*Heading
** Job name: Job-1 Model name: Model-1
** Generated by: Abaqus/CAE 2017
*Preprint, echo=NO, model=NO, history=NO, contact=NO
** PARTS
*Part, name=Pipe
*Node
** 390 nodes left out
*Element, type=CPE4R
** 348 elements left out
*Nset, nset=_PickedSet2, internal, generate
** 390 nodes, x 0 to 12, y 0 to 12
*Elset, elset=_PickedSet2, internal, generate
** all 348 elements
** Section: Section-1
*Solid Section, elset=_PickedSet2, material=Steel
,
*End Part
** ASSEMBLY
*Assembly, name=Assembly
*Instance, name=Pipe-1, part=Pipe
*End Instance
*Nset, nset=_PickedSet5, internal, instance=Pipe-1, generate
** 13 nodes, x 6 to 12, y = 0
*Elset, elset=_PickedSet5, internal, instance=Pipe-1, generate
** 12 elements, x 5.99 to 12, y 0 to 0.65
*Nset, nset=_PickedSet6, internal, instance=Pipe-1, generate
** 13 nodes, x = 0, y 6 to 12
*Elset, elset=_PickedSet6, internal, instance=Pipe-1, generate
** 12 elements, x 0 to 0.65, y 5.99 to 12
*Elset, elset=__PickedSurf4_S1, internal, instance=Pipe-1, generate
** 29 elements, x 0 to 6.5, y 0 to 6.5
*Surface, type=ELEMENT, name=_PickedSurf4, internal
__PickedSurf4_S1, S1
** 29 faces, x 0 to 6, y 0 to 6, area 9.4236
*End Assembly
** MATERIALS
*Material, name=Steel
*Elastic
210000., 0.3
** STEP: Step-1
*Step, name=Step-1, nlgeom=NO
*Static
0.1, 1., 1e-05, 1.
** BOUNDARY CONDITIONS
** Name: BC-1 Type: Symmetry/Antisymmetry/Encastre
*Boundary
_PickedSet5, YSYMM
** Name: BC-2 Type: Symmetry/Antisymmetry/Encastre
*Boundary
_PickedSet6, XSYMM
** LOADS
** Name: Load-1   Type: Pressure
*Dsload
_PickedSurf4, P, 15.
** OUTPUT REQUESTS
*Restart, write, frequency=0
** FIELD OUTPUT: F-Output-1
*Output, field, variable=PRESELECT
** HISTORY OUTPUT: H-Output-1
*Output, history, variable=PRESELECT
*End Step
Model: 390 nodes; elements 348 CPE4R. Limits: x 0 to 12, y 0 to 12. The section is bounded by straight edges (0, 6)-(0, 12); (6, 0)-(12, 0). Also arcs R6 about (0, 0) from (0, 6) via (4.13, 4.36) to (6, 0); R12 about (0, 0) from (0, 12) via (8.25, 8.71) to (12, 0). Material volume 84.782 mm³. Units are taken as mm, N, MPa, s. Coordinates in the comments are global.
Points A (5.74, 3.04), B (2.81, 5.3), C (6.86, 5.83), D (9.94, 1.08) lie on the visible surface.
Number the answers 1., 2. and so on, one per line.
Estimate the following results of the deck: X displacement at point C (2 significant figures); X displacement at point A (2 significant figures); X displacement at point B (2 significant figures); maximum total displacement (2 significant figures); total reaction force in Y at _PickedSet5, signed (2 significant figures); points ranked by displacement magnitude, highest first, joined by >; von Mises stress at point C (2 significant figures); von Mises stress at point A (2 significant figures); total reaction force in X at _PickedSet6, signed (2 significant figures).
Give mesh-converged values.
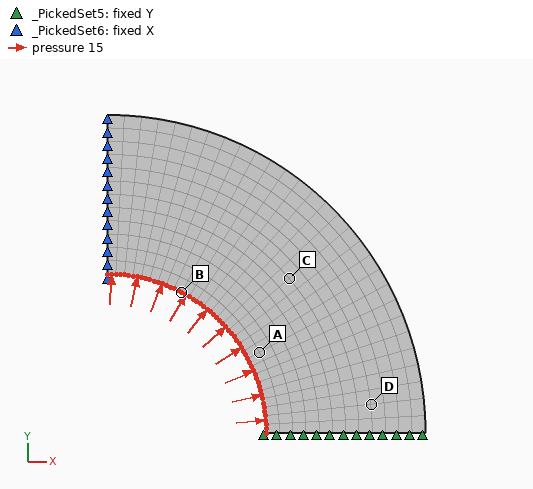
1. 4.6e-04 mm
2. 6.8e-04 mm
3. 3.8e-04 mm
4. 8.2e-04 mm
5. -90 N
6. B > A > C > D
7. 16 MPa
8. 30 MPa
9. -90 N
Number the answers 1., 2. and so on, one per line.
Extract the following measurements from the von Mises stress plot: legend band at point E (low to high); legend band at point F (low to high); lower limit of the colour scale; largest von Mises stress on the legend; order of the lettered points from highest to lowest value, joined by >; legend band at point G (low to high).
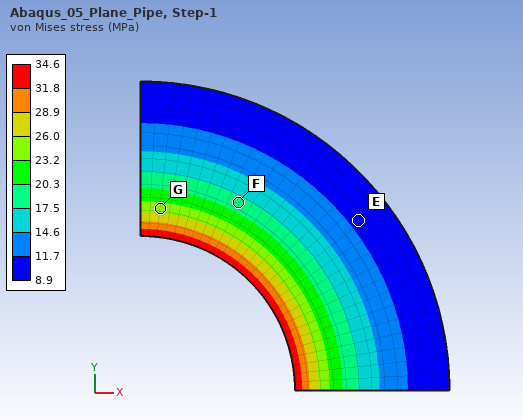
1. 8.9 to 11.7 MPa
2. 17.5 to 20.3 MPa
3. 8.9 MPa
4. 34.6 MPa
5. G > F > E
6. 23.2 to 26.0 MPa
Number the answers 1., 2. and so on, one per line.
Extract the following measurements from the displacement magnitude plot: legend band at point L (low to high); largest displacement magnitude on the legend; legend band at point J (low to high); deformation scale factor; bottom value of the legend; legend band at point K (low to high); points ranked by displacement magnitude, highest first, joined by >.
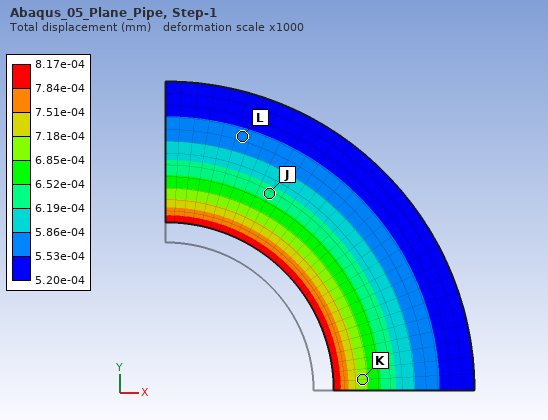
1. 5.53e-04 to 5.86e-04 mm
2. 8.17e-04 mm
3. 6.19e-04 to 6.52e-04 mm
4. 1000
5. 5.20e-04 mm
6. 6.85e-04 to 7.18e-04 mm
7. K > J > L
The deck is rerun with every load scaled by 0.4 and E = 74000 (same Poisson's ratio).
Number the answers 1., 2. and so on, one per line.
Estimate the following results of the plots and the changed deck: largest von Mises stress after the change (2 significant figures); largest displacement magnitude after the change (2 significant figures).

1. 14 MPa
2. 9.3e-04 mm
